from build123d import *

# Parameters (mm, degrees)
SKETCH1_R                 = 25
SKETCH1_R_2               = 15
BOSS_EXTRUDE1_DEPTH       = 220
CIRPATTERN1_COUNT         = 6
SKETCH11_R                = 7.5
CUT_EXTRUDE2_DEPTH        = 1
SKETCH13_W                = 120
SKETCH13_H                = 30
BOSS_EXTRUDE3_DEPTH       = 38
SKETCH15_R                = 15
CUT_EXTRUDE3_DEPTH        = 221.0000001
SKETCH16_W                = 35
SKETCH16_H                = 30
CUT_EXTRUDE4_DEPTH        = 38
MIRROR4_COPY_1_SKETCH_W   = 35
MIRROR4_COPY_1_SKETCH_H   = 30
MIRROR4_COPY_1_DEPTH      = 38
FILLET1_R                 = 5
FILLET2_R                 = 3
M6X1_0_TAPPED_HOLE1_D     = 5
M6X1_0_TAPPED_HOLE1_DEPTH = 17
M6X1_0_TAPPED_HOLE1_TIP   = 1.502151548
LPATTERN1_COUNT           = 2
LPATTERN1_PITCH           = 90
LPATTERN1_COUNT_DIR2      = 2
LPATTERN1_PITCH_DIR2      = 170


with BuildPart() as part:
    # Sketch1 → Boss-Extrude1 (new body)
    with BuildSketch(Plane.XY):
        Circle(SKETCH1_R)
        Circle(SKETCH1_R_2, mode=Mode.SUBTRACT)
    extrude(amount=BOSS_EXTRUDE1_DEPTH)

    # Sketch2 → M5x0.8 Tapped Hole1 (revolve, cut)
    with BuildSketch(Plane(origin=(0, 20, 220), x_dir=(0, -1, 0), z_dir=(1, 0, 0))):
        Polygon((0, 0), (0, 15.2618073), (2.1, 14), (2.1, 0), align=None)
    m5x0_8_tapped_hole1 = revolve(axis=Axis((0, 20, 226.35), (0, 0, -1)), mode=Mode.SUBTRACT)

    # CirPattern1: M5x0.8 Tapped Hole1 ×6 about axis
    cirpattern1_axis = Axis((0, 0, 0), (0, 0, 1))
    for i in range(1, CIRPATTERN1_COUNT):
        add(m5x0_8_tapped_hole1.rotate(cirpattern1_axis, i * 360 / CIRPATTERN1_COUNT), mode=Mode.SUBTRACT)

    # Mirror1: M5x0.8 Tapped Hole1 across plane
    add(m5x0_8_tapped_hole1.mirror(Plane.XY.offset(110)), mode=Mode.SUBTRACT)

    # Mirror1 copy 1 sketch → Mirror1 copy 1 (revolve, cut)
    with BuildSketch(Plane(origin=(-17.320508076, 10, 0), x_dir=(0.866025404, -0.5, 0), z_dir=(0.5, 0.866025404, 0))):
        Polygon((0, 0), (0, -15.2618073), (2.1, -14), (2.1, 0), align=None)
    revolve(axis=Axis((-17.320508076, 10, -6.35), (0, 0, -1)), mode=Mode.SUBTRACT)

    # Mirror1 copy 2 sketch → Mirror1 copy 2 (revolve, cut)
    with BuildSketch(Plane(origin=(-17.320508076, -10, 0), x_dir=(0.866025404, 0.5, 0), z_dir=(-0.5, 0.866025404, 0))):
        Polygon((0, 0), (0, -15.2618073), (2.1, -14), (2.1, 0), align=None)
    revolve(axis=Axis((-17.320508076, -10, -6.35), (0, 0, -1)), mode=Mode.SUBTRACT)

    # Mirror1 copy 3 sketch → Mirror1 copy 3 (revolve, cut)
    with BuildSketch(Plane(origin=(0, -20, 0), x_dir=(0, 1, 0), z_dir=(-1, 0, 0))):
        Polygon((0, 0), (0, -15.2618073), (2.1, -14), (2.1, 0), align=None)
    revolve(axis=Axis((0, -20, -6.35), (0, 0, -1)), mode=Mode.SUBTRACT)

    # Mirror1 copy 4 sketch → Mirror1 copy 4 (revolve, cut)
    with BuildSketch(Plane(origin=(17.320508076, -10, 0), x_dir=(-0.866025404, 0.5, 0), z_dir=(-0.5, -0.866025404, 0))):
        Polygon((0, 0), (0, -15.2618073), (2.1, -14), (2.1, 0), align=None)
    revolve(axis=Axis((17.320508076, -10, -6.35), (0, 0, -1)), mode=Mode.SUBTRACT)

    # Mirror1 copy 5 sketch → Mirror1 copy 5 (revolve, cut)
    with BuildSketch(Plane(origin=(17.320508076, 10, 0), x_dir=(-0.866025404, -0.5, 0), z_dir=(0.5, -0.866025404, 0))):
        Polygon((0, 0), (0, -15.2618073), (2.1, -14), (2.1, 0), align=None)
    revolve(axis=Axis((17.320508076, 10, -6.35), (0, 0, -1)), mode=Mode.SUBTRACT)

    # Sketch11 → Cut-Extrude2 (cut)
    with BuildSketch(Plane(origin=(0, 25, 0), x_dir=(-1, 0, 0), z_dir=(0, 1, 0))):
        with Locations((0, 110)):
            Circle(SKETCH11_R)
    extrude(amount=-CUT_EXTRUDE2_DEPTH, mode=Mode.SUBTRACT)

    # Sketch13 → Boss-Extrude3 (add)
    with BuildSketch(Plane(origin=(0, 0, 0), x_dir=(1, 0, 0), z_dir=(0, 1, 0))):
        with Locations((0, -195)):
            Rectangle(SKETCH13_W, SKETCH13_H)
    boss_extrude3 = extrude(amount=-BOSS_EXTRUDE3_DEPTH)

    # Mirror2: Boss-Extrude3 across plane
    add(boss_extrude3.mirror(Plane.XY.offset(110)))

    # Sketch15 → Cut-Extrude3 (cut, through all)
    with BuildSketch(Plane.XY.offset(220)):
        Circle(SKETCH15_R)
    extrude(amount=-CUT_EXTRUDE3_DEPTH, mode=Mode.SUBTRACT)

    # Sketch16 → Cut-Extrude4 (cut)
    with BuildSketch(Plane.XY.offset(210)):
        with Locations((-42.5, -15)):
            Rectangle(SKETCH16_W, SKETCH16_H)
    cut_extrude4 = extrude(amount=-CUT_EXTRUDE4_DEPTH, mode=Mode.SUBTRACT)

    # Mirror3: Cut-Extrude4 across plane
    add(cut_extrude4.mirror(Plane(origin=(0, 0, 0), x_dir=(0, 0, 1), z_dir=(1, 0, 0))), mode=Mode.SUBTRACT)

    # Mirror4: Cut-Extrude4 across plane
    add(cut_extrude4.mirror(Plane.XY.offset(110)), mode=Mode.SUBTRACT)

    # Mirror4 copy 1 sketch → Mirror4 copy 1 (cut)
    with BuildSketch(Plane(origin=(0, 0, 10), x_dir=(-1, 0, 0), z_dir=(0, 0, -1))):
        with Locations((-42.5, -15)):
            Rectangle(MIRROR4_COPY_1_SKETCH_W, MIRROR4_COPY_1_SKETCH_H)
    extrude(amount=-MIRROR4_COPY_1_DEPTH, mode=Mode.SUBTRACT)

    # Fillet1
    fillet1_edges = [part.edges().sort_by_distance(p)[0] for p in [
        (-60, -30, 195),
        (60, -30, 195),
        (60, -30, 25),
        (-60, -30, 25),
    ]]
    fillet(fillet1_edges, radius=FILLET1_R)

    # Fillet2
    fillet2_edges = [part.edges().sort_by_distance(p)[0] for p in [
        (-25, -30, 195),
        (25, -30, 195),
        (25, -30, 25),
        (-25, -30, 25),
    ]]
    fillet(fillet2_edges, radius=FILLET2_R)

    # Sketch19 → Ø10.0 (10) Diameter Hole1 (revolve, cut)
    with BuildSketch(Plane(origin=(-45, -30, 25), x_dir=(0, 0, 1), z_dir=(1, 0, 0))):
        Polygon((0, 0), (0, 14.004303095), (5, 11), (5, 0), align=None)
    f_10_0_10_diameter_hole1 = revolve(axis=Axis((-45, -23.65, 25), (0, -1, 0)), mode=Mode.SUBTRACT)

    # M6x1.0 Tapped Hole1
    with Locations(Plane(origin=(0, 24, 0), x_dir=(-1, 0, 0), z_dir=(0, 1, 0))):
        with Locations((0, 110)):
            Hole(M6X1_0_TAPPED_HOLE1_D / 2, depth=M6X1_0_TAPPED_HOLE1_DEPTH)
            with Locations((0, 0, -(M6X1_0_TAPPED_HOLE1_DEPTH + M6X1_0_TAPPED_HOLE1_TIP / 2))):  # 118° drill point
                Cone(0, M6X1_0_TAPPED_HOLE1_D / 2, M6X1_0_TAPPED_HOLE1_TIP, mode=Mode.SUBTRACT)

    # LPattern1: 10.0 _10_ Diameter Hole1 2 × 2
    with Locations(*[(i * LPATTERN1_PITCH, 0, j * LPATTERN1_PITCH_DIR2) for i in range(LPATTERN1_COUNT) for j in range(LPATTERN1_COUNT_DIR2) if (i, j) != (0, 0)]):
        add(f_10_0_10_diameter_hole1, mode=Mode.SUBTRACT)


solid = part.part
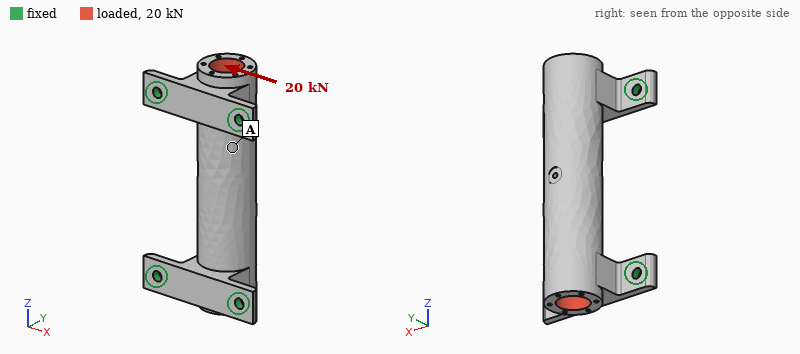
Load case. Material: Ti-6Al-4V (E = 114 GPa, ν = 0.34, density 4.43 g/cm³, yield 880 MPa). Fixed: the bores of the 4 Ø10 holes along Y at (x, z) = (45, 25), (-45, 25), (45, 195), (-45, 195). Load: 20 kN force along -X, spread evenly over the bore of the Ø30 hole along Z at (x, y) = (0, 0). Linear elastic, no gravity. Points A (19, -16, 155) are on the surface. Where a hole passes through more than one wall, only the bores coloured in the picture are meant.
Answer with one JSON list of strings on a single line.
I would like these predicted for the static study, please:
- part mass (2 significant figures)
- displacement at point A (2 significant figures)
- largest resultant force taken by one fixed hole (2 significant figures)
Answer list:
["1.6 kg", "0.049 mm", "7.2 kN"]
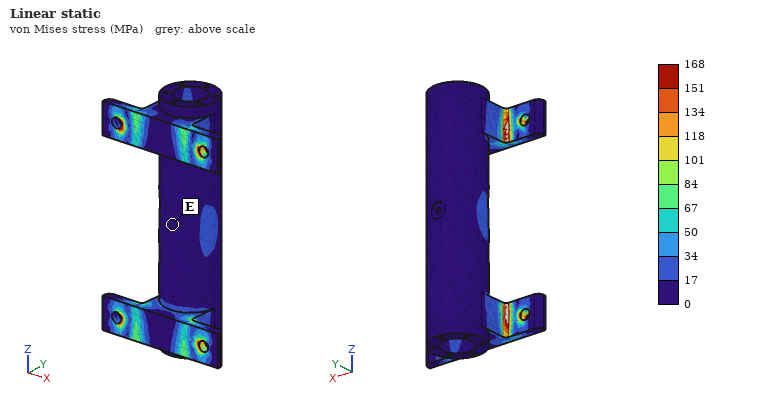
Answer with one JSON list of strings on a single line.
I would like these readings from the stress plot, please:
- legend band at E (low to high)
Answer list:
["0 to 17 MPa"]
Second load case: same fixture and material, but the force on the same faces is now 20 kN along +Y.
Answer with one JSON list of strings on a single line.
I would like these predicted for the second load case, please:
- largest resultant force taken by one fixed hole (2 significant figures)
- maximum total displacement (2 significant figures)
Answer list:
["5.9 kN", "65 µm"]
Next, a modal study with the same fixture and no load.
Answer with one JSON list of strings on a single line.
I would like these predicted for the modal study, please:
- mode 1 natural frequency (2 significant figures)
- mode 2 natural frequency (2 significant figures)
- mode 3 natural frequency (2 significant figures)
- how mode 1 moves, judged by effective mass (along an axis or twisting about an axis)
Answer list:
["2300 Hz", "2600 Hz", "2700 Hz", "along X"]
